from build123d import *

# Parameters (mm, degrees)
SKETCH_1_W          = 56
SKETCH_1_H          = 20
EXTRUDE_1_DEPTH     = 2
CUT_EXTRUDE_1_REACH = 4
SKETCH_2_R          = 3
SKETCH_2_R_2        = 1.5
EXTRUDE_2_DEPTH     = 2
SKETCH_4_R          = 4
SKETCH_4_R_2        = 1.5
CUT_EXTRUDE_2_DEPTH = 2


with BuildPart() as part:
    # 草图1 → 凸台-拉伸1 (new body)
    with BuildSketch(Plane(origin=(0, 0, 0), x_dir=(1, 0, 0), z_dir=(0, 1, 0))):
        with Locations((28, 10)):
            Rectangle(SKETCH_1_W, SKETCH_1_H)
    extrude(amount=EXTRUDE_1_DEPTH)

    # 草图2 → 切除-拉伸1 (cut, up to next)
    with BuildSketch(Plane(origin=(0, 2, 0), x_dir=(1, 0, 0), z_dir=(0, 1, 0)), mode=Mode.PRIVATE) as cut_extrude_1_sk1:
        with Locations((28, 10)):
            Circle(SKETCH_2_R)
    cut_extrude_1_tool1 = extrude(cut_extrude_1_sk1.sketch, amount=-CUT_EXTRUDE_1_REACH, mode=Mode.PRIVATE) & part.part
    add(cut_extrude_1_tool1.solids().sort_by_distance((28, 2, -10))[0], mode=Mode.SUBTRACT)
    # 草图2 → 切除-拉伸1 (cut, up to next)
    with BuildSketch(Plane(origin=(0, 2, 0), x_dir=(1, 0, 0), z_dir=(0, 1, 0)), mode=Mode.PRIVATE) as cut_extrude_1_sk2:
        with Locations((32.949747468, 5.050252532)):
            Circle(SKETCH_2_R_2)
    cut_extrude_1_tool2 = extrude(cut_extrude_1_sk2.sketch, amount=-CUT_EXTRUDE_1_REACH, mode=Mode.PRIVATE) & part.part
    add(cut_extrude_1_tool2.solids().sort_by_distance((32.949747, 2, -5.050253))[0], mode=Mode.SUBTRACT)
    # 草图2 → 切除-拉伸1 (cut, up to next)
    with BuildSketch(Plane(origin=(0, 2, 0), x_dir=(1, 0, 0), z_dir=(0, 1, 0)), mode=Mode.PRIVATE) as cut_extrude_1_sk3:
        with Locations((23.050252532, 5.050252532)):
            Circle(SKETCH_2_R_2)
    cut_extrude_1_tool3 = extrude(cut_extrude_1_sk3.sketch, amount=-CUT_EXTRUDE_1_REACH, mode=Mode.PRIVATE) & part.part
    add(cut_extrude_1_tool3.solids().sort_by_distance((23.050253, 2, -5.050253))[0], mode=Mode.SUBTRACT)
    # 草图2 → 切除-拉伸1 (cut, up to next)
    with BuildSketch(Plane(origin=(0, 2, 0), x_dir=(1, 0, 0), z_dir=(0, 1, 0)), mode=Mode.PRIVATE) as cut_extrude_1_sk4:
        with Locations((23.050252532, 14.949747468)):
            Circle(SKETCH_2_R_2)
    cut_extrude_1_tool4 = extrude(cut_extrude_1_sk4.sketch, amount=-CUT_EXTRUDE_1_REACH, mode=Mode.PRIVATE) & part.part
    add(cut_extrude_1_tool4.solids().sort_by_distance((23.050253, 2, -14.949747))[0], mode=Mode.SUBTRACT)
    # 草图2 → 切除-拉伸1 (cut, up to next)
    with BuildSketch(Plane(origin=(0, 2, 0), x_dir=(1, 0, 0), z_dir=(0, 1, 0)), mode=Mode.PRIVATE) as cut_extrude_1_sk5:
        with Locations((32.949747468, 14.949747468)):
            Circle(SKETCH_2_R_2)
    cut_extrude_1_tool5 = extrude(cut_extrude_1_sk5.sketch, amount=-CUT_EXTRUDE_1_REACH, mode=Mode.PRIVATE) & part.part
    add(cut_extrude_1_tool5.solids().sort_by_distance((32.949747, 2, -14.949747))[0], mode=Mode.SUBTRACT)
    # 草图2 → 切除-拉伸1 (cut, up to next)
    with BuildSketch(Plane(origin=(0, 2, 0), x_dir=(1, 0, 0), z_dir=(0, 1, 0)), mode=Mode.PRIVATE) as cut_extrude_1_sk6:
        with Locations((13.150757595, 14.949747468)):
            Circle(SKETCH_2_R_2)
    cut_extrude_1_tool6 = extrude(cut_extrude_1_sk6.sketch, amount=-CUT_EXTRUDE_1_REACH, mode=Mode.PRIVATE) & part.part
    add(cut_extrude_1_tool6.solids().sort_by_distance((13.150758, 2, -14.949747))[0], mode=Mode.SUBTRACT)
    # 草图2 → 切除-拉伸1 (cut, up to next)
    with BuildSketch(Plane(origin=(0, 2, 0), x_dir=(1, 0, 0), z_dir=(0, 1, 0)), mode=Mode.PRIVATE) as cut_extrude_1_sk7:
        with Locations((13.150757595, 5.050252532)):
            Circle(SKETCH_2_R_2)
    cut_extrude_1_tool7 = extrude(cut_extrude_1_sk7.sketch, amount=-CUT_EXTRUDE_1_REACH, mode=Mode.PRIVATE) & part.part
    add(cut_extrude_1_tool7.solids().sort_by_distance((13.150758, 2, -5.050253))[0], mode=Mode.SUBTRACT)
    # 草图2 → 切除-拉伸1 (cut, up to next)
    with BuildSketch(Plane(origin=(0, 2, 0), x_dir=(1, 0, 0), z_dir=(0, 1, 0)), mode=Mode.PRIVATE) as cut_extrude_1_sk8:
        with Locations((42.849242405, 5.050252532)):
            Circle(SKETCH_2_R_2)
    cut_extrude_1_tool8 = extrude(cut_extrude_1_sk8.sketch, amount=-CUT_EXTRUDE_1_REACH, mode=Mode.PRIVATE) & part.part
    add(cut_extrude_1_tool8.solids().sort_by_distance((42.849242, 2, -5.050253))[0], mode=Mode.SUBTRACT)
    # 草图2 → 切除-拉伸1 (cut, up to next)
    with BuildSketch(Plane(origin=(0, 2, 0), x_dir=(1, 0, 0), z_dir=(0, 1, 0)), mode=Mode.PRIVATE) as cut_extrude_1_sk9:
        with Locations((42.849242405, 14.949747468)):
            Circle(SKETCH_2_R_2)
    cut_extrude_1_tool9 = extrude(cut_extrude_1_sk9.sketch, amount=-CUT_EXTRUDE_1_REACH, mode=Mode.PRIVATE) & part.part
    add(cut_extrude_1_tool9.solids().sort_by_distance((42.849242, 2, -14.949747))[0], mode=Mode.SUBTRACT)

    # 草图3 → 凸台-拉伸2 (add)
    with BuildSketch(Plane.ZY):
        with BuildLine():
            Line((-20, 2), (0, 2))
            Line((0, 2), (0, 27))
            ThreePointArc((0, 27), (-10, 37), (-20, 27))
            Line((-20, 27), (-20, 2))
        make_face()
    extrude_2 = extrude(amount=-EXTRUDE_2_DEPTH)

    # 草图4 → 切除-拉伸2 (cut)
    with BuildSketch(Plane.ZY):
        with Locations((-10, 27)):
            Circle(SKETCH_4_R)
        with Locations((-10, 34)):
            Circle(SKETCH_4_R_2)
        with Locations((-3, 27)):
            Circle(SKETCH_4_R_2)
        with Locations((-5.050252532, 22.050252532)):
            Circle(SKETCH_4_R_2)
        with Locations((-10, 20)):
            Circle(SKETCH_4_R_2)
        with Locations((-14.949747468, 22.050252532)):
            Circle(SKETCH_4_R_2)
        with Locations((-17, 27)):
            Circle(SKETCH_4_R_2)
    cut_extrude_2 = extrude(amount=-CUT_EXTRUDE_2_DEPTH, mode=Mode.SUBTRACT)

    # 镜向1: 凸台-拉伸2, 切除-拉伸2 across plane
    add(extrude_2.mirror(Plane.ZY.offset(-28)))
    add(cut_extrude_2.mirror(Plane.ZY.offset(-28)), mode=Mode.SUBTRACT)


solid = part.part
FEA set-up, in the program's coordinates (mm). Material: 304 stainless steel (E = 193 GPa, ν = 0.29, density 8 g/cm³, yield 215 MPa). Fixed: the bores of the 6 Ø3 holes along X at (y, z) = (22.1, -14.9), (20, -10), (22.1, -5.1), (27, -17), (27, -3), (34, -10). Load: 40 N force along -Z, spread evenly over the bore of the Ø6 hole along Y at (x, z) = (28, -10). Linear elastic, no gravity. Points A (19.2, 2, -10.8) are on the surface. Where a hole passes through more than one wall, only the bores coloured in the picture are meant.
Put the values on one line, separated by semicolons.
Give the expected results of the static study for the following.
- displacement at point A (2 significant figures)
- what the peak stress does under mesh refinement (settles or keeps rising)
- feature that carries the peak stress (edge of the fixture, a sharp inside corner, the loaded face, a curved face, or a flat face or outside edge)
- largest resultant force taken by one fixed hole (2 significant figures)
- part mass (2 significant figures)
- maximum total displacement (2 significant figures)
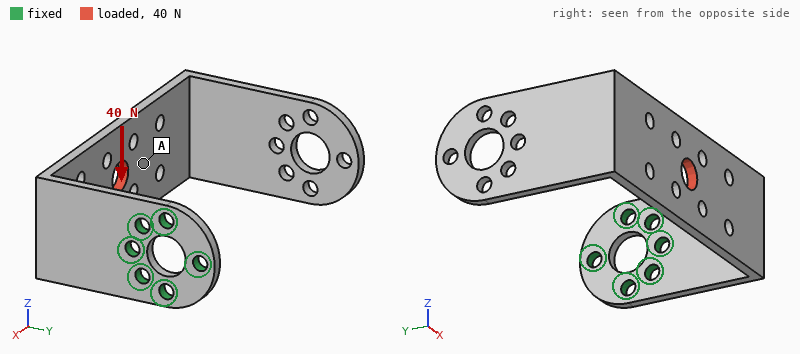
0.14 mm; keeps rising; edge of the fixture; 84 N; 35 g; 0.24 mm
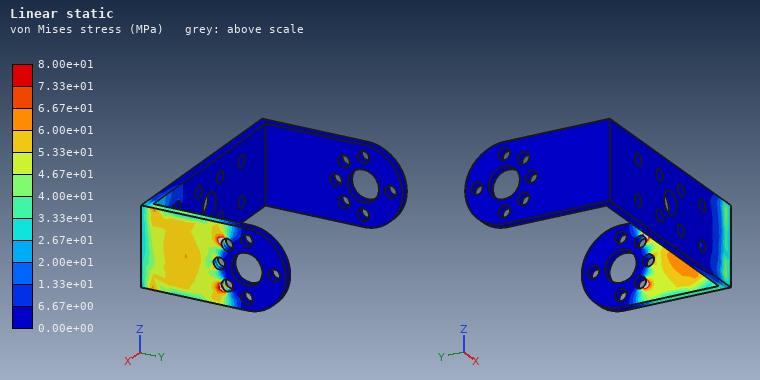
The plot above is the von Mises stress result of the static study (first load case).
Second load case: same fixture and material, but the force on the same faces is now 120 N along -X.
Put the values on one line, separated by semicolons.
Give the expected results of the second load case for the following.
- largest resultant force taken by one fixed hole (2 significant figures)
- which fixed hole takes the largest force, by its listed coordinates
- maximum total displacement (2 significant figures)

210 N; (20, -10); 0.47 mm
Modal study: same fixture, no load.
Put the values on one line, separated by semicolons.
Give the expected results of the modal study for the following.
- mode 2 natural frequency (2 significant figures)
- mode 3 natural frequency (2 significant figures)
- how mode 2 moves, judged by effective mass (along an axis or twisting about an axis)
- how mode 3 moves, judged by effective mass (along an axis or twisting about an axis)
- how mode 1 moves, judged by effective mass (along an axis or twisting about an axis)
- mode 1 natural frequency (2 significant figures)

360 Hz; 730 Hz; along Z; along X; along Y; 200 Hz
